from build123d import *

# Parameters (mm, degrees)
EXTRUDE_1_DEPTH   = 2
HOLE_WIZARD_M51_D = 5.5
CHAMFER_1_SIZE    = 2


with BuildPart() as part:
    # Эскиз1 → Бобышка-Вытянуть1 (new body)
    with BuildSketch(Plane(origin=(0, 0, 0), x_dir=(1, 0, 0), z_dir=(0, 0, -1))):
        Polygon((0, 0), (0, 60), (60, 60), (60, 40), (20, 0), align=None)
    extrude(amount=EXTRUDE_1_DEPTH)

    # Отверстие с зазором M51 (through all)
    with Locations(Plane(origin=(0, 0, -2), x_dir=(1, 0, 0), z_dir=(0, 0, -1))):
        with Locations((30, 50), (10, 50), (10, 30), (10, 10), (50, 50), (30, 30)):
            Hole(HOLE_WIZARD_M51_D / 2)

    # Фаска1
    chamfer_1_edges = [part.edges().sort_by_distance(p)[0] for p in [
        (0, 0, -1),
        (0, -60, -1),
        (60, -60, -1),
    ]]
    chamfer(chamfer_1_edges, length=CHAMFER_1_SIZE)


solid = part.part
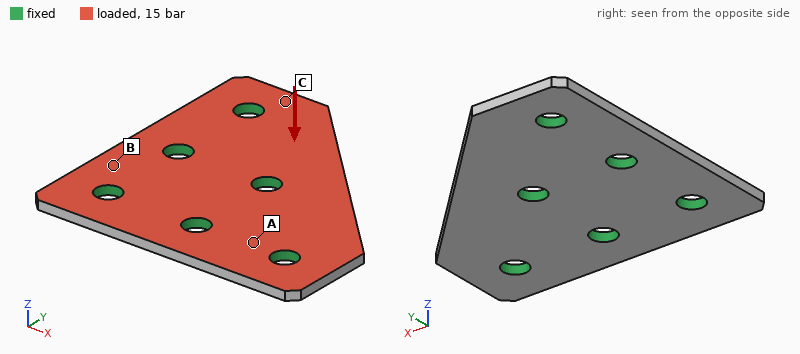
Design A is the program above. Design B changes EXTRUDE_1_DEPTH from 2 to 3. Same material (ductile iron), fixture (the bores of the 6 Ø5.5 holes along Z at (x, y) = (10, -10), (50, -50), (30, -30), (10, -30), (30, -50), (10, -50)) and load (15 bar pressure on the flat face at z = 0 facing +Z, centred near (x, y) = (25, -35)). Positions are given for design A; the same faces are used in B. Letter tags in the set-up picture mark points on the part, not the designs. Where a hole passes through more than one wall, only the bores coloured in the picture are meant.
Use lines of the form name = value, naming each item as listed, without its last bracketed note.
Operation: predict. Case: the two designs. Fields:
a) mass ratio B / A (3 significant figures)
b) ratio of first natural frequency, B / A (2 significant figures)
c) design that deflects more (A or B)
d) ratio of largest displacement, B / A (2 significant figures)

mass ratio B / A = 1.50
ratio of first natural frequency, B / A = 1.4
design that deflects more = A
ratio of largest displacement, B / A = 0.32
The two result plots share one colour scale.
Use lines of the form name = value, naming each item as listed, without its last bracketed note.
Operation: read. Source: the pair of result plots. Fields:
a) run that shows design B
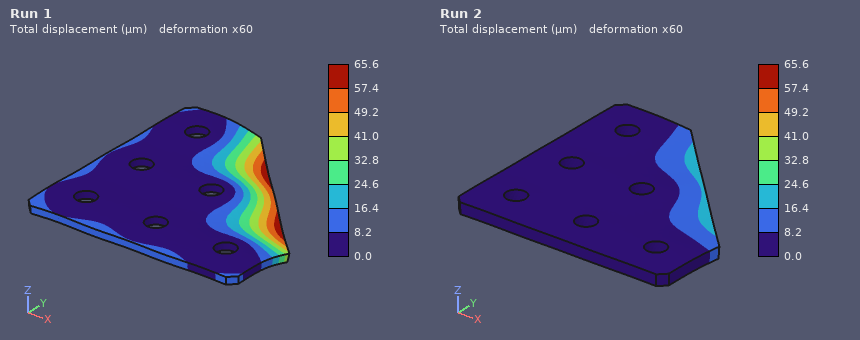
run that shows design B = Run 2
